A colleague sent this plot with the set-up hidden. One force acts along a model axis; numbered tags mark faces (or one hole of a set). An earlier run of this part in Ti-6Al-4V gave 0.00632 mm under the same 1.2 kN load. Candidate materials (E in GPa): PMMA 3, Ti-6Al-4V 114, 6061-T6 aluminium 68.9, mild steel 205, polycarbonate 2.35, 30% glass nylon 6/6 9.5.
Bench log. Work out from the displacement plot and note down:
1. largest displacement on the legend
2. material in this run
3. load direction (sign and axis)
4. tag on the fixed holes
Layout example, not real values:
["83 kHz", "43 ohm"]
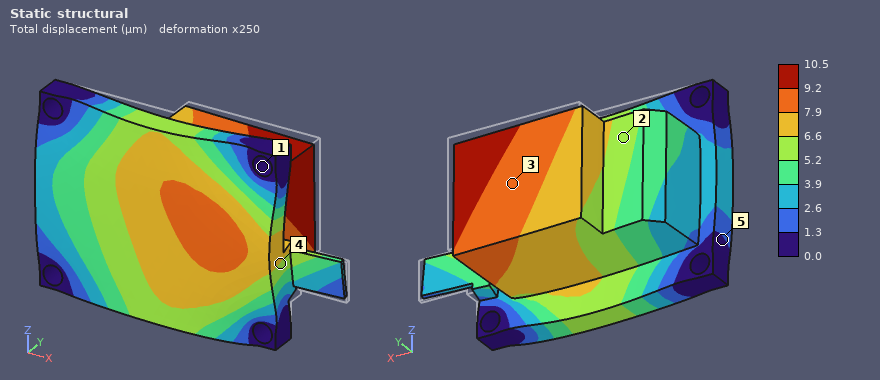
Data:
["10.5 µm", "6061-T6 aluminium", "-Y", "1"]
